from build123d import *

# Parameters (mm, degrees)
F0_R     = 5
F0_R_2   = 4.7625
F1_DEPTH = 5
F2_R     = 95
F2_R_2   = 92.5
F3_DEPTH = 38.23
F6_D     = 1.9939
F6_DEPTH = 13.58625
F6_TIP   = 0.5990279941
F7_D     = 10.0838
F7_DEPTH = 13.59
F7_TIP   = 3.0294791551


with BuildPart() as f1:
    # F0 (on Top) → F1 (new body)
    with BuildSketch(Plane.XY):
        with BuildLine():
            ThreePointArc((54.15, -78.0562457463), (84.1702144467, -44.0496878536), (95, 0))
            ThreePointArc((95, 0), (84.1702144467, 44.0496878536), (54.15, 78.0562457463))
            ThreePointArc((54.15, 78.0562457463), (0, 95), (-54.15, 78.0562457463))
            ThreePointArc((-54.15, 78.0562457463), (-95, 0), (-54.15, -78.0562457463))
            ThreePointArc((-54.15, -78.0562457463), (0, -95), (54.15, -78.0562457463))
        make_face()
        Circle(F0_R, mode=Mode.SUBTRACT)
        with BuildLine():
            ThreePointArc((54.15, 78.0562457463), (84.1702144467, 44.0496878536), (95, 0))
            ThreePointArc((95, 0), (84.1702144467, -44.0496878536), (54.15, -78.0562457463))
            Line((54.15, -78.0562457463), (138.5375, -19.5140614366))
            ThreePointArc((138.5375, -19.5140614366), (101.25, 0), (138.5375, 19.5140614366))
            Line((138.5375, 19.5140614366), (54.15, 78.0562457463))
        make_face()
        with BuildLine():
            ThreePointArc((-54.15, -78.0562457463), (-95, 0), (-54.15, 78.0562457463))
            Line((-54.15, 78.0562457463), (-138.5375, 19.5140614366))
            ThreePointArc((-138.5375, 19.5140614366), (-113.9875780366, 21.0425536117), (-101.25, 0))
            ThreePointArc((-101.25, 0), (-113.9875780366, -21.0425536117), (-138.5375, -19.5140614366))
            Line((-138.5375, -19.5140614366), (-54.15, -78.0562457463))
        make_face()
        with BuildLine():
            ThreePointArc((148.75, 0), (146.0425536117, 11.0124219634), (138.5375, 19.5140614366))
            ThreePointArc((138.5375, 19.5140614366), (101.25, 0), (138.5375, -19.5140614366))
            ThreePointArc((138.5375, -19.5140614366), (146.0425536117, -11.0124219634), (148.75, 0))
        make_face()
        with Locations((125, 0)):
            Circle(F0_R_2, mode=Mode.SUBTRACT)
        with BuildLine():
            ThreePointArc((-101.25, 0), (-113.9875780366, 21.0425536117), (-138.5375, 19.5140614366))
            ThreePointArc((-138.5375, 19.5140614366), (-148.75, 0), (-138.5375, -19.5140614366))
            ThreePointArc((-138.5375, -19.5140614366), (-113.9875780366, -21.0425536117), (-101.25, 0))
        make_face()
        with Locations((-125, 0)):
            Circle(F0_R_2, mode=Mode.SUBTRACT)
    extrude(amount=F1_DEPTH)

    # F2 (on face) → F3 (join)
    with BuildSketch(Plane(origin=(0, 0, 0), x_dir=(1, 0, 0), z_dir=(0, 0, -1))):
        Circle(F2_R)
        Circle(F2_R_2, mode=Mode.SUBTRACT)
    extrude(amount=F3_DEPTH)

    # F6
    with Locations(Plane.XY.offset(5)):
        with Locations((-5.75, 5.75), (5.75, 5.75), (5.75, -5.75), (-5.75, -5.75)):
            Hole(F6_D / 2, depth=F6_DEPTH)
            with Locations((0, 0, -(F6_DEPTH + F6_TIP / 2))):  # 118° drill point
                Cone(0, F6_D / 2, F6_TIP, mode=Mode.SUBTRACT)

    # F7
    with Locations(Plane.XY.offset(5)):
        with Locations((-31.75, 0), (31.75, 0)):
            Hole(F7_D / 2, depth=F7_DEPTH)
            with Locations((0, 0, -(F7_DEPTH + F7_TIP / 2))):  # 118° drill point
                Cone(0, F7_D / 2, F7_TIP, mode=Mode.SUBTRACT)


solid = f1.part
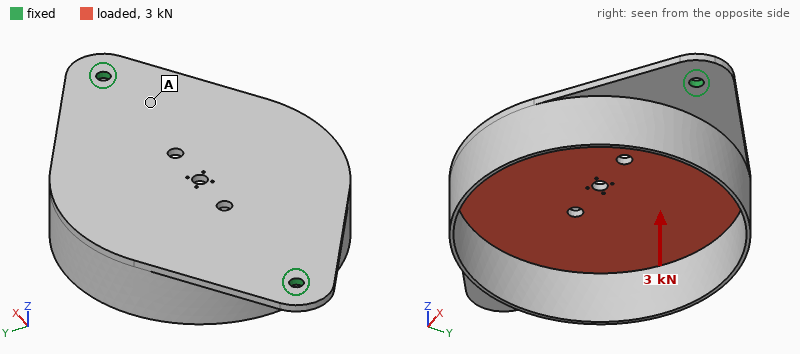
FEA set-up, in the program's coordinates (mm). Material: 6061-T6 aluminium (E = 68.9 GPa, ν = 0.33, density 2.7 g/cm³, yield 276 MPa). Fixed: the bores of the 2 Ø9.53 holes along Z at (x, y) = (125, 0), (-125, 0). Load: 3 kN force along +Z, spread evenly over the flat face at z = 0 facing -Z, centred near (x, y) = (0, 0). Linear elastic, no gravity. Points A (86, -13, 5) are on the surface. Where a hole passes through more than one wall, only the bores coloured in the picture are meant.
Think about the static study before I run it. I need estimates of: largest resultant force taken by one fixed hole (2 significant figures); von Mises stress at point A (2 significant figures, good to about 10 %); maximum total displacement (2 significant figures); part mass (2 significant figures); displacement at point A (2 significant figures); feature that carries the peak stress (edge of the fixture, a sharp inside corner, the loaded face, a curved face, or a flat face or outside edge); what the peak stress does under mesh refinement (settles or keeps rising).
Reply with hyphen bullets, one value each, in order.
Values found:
- 1.6 kN
- 31 MPa
- 1.8 mm
- 640 g
- 0.53 mm
- edge of the fixture
- keeps rising
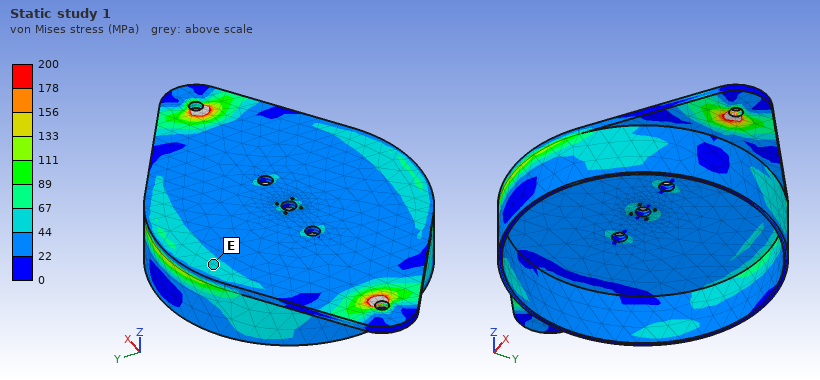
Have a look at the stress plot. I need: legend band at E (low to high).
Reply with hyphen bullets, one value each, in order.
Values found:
- 44 to 67 MPa
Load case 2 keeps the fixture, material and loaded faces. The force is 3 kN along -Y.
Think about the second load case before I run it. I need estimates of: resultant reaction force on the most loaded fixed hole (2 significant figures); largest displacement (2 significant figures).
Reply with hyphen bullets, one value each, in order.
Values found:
- 1.5 kN
- 0.19 mm
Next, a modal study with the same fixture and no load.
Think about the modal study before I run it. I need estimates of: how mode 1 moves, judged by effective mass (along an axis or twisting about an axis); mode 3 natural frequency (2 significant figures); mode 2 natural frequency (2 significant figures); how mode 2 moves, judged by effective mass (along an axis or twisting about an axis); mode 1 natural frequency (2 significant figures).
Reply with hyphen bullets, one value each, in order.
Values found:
- twisting about X
- 890 Hz
- 340 Hz
- along Z
- 260 Hz
